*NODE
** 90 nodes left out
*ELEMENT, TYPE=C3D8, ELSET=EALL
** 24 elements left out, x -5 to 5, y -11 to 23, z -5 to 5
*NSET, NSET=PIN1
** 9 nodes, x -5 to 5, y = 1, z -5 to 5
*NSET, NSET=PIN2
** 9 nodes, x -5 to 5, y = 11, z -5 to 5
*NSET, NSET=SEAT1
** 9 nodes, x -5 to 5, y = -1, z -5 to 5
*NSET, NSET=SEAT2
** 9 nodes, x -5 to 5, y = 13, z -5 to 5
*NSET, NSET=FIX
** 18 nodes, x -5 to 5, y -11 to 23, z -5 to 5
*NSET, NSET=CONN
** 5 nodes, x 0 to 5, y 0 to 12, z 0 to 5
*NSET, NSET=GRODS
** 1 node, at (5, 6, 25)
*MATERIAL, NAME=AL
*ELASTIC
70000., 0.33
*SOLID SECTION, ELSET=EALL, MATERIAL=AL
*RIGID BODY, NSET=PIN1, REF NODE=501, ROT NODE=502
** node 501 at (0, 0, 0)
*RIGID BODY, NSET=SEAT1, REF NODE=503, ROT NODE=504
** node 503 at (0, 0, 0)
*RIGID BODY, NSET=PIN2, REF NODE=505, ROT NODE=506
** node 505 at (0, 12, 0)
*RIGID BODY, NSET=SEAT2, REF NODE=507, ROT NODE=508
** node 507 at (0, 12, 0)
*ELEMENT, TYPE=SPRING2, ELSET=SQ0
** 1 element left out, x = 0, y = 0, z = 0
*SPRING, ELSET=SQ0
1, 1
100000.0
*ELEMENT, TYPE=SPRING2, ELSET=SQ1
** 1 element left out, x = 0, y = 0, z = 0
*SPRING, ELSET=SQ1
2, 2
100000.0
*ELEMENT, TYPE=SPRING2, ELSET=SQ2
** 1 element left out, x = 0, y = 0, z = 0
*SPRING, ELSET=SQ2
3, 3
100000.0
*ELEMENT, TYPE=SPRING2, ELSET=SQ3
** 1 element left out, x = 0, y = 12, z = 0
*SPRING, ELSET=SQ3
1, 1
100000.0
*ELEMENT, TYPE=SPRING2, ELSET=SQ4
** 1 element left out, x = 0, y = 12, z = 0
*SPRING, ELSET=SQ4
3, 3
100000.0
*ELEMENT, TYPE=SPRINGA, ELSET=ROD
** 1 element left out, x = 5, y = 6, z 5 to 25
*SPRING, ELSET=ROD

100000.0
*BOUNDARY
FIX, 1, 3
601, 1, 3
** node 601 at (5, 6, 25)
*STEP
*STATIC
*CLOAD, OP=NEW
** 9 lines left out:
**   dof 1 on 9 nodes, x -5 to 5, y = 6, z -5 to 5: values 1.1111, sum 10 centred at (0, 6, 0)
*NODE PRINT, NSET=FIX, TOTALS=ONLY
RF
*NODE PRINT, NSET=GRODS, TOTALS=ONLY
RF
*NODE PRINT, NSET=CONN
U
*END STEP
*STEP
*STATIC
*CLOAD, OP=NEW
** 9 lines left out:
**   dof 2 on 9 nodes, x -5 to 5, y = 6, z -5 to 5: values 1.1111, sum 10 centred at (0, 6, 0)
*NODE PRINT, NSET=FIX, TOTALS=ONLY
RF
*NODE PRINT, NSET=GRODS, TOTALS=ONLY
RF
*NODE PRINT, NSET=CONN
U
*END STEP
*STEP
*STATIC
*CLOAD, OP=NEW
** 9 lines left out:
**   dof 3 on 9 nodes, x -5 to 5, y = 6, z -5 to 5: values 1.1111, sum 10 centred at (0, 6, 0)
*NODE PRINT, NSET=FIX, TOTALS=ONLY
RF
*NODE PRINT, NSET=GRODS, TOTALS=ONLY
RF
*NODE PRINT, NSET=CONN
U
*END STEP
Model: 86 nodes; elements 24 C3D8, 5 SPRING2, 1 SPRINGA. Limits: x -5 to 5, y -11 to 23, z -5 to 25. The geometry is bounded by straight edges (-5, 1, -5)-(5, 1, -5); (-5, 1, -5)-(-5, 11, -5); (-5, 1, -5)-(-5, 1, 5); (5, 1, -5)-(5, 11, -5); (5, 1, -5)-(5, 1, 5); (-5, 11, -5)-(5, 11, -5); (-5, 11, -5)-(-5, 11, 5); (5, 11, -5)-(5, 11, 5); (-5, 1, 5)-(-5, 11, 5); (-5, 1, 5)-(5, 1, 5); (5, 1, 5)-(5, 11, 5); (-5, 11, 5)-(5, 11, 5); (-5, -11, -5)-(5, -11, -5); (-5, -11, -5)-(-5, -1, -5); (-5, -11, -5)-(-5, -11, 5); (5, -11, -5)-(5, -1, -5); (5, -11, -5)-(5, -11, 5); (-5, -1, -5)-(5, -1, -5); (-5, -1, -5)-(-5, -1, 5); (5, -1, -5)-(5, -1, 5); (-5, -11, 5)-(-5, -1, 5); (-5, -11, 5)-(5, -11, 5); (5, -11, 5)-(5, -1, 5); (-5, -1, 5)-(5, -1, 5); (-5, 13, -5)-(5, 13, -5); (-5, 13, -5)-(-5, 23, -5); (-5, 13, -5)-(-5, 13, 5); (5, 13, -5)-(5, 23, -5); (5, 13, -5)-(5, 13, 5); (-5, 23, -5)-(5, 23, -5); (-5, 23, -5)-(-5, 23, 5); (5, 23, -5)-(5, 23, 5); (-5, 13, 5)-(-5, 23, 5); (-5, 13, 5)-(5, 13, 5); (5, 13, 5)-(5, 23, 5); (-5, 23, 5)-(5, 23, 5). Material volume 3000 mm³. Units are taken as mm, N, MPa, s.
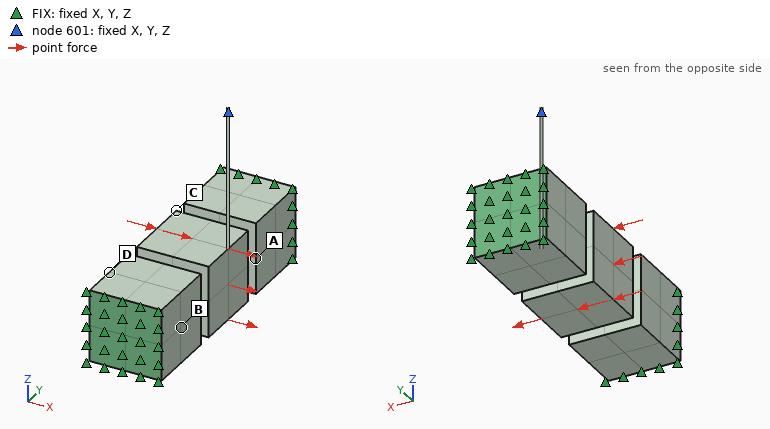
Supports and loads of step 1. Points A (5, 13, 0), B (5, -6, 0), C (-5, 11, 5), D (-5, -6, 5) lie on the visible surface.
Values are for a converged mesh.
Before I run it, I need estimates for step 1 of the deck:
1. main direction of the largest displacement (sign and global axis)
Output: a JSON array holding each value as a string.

["+X"]
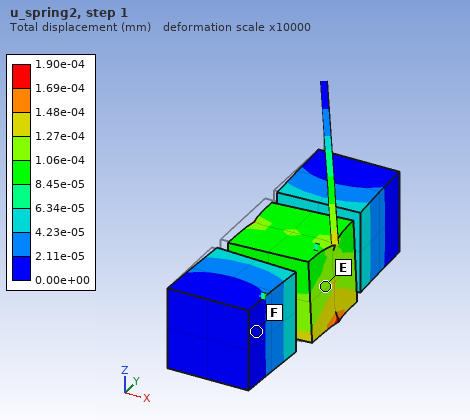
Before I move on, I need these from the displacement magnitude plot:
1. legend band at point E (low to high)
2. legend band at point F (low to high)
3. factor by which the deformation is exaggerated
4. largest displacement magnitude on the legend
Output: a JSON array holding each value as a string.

["1.06e-04 to 1.27e-04 mm", "0.00e+00 to 2.11e-05 mm", "10000", "1.90e-04 mm"]
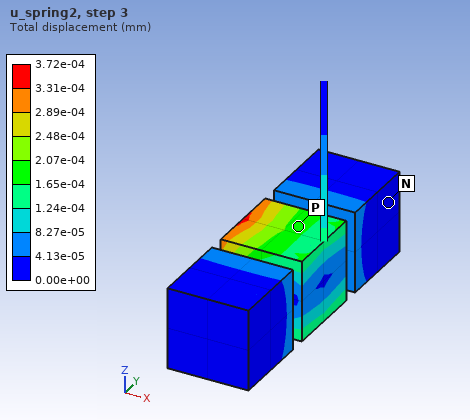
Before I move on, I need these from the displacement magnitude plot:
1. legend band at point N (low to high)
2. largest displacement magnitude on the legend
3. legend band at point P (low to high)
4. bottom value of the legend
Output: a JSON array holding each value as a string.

["0.00e+00 to 4.13e-05 mm", "3.72e-04 mm", "1.65e-04 to 2.07e-04 mm", "0.00e+00 mm"]
